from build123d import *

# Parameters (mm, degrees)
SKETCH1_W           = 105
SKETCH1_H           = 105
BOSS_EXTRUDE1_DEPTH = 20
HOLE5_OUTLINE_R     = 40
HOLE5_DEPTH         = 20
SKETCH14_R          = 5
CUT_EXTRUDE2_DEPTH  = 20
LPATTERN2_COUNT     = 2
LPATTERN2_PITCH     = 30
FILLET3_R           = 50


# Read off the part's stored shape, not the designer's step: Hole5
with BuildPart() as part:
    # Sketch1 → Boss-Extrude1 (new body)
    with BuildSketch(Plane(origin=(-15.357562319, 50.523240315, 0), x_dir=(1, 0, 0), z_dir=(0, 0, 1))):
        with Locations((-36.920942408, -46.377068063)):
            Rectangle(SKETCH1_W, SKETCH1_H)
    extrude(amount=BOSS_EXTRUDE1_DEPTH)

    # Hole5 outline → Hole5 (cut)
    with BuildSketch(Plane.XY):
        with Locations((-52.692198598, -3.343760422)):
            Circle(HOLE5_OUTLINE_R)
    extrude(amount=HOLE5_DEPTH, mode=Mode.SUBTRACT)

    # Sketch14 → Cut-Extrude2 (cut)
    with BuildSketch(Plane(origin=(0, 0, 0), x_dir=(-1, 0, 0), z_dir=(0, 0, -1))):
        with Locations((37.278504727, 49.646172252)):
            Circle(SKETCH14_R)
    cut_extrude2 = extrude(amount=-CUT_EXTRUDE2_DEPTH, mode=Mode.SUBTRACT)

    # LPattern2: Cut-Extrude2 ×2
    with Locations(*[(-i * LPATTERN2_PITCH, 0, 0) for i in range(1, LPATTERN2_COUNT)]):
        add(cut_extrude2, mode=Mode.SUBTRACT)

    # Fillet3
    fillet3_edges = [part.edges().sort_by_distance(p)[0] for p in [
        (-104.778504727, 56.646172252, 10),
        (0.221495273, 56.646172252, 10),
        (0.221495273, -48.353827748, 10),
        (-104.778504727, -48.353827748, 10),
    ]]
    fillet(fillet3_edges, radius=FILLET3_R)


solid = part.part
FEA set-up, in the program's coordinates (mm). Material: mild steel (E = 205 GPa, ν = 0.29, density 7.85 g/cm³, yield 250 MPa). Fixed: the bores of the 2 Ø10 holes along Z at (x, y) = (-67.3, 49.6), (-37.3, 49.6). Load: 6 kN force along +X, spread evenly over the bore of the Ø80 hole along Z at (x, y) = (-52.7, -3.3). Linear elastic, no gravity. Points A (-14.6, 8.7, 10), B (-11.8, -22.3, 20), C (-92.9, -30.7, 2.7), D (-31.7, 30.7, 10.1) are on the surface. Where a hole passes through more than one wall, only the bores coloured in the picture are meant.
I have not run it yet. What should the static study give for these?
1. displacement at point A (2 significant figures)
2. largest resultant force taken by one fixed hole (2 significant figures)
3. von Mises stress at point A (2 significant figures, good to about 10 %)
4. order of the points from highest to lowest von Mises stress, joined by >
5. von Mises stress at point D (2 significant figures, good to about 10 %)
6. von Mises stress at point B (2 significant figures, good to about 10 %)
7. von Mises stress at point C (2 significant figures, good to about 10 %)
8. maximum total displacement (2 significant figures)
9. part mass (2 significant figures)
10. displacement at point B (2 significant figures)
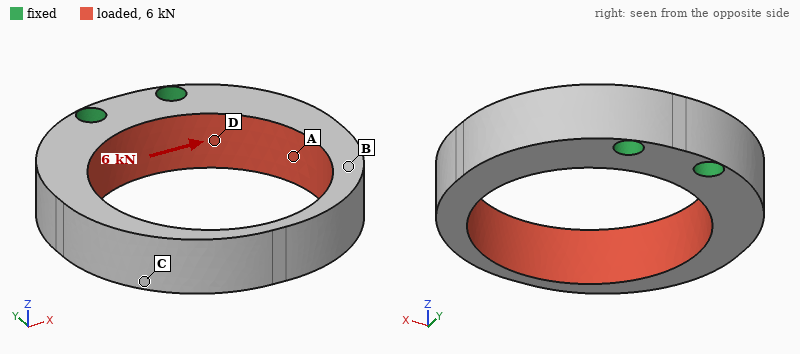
0.053 mm
5.8 kN
60 MPa
D > A > C > B
100 MPa
16 MPa
39 MPa
0.17 mm
580 g
0.13 mm
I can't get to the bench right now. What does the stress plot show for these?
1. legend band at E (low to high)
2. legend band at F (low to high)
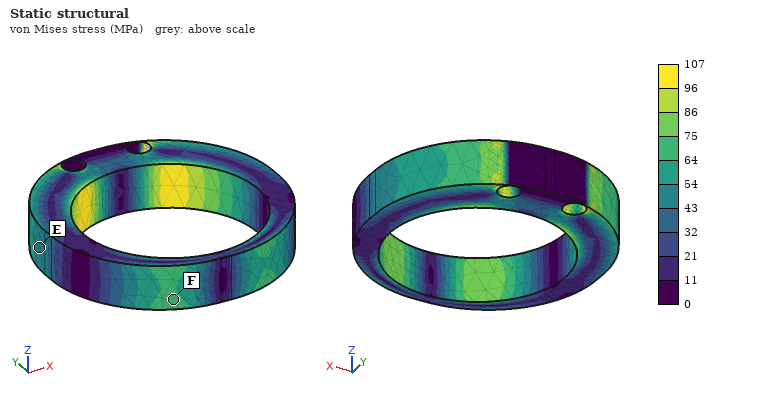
43 to 54 MPa
64 to 75 MPa
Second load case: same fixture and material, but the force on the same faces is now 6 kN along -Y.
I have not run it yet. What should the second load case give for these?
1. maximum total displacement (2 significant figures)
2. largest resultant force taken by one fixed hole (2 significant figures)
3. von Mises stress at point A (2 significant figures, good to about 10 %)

46 µm
3.6 kN
22 MPa
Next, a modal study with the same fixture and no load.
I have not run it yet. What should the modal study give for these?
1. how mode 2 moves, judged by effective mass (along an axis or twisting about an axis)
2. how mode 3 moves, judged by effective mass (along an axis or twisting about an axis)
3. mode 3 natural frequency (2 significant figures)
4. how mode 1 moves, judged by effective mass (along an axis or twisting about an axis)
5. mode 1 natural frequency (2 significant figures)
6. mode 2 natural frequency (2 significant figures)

along X
twisting about Y
2800 Hz
along Z
1500 Hz
1800 Hz
